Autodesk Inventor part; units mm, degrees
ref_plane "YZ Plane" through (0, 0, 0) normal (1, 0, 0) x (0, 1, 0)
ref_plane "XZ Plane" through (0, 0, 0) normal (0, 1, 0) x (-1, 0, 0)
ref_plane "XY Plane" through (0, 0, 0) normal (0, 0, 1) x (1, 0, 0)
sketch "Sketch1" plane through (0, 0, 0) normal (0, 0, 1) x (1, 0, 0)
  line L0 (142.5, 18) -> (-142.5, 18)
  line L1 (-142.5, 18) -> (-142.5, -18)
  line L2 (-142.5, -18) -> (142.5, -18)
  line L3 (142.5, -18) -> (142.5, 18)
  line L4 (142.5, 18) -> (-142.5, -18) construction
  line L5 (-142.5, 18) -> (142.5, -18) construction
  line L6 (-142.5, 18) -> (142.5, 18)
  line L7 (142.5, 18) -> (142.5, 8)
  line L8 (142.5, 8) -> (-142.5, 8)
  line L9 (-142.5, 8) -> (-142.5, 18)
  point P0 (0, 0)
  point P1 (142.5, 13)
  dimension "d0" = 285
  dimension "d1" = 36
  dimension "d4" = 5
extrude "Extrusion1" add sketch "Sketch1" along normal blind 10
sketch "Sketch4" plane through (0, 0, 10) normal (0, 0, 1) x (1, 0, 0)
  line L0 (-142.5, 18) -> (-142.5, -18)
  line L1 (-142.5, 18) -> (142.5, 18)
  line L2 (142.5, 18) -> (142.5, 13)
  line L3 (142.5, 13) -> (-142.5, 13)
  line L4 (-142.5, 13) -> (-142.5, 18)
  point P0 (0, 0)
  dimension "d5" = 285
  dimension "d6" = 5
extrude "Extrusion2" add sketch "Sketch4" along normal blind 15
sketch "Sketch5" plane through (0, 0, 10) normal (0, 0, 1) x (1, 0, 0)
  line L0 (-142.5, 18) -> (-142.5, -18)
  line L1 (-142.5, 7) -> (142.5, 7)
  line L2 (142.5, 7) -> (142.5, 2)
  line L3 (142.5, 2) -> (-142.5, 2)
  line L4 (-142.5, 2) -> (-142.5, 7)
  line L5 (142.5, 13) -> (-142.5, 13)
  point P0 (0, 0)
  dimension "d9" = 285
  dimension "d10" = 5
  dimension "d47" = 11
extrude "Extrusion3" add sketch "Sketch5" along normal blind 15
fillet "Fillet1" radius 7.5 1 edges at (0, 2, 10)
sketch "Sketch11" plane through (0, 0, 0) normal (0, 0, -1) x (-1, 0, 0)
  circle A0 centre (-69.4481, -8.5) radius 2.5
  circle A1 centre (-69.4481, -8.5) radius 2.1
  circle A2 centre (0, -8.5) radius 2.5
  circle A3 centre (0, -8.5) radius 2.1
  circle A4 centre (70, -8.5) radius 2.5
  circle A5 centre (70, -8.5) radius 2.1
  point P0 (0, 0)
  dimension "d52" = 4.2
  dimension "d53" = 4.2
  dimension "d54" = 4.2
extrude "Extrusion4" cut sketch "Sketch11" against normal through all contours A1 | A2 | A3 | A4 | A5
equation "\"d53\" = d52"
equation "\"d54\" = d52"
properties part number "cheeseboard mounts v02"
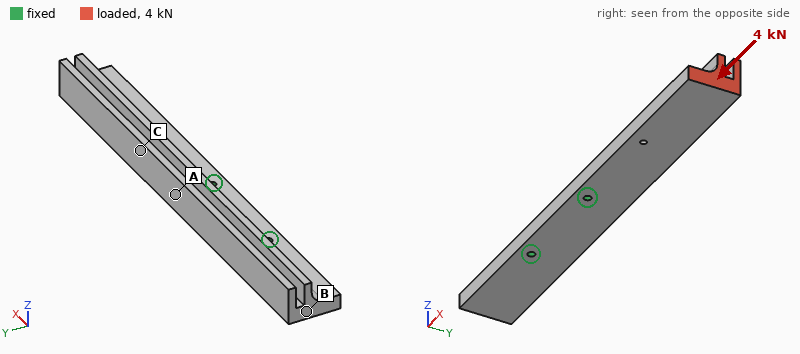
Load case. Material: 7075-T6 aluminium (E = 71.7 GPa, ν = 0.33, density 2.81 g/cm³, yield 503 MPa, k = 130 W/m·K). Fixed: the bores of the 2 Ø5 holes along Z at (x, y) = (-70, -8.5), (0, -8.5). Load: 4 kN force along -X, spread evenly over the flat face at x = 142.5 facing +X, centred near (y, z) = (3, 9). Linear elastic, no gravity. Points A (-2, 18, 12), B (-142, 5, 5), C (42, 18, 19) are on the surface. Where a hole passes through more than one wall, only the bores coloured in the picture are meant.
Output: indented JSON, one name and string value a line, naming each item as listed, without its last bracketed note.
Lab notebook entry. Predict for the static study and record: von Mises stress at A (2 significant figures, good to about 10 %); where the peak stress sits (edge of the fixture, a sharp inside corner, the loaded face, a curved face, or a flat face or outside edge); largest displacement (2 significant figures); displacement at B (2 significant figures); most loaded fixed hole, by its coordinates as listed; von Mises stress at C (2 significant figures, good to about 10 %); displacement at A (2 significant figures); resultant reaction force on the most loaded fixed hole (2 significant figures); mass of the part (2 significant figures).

{
  "von Mises stress at A": "9.0 MPa",
  "where the peak stress sits": "edge of the fixture",
  "largest displacement": "40 µm",
  "displacement at B": "7.3 µm",
  "most loaded fixed hole, by its coordinates as listed": "(0, -8.5)",
  "von Mises stress at C": "7.7 MPa",
  "displacement at A": "7.1 µm",
  "resultant reaction force on the most loaded fixed hole": "2.9 kN",
  "mass of the part": "420 g"
}
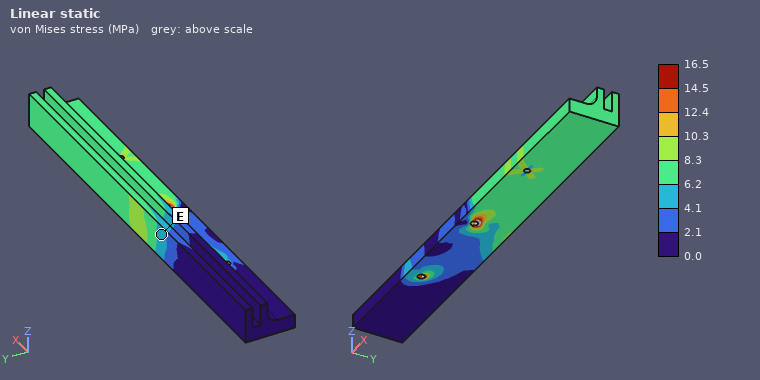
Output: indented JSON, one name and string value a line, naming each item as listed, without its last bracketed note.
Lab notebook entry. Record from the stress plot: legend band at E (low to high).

{
  "legend band at E": "4.1 to 6.2 MPa"
}
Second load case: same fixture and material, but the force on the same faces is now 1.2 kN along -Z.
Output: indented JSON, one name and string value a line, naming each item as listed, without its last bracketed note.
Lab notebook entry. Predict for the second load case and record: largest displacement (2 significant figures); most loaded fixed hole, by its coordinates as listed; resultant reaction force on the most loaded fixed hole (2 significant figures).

{
  "largest displacement": "1.3 mm",
  "most loaded fixed hole, by its coordinates as listed": "(0, -8.5)",
  "resultant reaction force on the most loaded fixed hole": "3.1 kN"
}
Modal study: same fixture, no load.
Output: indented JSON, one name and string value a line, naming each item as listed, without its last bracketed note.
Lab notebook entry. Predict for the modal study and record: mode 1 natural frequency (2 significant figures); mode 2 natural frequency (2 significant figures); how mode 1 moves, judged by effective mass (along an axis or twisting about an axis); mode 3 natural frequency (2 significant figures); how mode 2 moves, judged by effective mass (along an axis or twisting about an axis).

{
  "mode 1 natural frequency": "630 Hz",
  "mode 2 natural frequency": "1100 Hz",
  "how mode 1 moves, judged by effective mass": "along Z",
  "mode 3 natural frequency": "1900 Hz",
  "how mode 2 moves, judged by effective mass": "along Y"
}
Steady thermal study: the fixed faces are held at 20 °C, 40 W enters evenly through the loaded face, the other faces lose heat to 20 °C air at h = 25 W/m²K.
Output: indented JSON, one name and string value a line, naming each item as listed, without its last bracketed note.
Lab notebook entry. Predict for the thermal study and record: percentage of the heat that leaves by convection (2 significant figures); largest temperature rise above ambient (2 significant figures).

{
  "percentage of the heat that leaves by convection": "44 %",
  "largest temperature rise above ambient": "65 K"
}
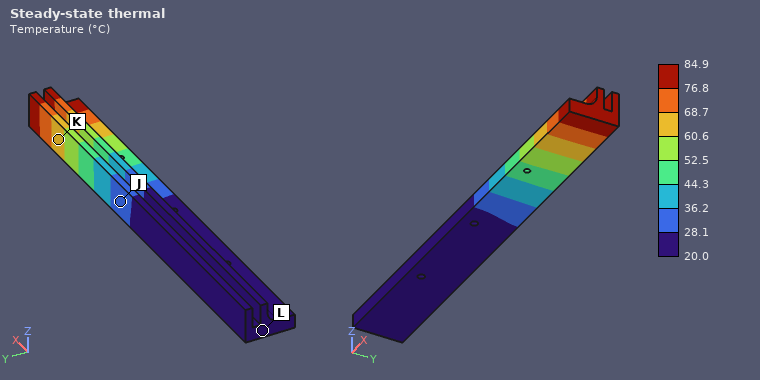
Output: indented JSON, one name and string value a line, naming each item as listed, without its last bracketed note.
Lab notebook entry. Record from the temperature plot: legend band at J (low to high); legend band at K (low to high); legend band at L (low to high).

{
  "legend band at J": "28.1 to 36.2 °C",
  "legend band at K": "60.6 to 68.7 °C",
  "legend band at L": "20.0 to 28.1 °C"
}
